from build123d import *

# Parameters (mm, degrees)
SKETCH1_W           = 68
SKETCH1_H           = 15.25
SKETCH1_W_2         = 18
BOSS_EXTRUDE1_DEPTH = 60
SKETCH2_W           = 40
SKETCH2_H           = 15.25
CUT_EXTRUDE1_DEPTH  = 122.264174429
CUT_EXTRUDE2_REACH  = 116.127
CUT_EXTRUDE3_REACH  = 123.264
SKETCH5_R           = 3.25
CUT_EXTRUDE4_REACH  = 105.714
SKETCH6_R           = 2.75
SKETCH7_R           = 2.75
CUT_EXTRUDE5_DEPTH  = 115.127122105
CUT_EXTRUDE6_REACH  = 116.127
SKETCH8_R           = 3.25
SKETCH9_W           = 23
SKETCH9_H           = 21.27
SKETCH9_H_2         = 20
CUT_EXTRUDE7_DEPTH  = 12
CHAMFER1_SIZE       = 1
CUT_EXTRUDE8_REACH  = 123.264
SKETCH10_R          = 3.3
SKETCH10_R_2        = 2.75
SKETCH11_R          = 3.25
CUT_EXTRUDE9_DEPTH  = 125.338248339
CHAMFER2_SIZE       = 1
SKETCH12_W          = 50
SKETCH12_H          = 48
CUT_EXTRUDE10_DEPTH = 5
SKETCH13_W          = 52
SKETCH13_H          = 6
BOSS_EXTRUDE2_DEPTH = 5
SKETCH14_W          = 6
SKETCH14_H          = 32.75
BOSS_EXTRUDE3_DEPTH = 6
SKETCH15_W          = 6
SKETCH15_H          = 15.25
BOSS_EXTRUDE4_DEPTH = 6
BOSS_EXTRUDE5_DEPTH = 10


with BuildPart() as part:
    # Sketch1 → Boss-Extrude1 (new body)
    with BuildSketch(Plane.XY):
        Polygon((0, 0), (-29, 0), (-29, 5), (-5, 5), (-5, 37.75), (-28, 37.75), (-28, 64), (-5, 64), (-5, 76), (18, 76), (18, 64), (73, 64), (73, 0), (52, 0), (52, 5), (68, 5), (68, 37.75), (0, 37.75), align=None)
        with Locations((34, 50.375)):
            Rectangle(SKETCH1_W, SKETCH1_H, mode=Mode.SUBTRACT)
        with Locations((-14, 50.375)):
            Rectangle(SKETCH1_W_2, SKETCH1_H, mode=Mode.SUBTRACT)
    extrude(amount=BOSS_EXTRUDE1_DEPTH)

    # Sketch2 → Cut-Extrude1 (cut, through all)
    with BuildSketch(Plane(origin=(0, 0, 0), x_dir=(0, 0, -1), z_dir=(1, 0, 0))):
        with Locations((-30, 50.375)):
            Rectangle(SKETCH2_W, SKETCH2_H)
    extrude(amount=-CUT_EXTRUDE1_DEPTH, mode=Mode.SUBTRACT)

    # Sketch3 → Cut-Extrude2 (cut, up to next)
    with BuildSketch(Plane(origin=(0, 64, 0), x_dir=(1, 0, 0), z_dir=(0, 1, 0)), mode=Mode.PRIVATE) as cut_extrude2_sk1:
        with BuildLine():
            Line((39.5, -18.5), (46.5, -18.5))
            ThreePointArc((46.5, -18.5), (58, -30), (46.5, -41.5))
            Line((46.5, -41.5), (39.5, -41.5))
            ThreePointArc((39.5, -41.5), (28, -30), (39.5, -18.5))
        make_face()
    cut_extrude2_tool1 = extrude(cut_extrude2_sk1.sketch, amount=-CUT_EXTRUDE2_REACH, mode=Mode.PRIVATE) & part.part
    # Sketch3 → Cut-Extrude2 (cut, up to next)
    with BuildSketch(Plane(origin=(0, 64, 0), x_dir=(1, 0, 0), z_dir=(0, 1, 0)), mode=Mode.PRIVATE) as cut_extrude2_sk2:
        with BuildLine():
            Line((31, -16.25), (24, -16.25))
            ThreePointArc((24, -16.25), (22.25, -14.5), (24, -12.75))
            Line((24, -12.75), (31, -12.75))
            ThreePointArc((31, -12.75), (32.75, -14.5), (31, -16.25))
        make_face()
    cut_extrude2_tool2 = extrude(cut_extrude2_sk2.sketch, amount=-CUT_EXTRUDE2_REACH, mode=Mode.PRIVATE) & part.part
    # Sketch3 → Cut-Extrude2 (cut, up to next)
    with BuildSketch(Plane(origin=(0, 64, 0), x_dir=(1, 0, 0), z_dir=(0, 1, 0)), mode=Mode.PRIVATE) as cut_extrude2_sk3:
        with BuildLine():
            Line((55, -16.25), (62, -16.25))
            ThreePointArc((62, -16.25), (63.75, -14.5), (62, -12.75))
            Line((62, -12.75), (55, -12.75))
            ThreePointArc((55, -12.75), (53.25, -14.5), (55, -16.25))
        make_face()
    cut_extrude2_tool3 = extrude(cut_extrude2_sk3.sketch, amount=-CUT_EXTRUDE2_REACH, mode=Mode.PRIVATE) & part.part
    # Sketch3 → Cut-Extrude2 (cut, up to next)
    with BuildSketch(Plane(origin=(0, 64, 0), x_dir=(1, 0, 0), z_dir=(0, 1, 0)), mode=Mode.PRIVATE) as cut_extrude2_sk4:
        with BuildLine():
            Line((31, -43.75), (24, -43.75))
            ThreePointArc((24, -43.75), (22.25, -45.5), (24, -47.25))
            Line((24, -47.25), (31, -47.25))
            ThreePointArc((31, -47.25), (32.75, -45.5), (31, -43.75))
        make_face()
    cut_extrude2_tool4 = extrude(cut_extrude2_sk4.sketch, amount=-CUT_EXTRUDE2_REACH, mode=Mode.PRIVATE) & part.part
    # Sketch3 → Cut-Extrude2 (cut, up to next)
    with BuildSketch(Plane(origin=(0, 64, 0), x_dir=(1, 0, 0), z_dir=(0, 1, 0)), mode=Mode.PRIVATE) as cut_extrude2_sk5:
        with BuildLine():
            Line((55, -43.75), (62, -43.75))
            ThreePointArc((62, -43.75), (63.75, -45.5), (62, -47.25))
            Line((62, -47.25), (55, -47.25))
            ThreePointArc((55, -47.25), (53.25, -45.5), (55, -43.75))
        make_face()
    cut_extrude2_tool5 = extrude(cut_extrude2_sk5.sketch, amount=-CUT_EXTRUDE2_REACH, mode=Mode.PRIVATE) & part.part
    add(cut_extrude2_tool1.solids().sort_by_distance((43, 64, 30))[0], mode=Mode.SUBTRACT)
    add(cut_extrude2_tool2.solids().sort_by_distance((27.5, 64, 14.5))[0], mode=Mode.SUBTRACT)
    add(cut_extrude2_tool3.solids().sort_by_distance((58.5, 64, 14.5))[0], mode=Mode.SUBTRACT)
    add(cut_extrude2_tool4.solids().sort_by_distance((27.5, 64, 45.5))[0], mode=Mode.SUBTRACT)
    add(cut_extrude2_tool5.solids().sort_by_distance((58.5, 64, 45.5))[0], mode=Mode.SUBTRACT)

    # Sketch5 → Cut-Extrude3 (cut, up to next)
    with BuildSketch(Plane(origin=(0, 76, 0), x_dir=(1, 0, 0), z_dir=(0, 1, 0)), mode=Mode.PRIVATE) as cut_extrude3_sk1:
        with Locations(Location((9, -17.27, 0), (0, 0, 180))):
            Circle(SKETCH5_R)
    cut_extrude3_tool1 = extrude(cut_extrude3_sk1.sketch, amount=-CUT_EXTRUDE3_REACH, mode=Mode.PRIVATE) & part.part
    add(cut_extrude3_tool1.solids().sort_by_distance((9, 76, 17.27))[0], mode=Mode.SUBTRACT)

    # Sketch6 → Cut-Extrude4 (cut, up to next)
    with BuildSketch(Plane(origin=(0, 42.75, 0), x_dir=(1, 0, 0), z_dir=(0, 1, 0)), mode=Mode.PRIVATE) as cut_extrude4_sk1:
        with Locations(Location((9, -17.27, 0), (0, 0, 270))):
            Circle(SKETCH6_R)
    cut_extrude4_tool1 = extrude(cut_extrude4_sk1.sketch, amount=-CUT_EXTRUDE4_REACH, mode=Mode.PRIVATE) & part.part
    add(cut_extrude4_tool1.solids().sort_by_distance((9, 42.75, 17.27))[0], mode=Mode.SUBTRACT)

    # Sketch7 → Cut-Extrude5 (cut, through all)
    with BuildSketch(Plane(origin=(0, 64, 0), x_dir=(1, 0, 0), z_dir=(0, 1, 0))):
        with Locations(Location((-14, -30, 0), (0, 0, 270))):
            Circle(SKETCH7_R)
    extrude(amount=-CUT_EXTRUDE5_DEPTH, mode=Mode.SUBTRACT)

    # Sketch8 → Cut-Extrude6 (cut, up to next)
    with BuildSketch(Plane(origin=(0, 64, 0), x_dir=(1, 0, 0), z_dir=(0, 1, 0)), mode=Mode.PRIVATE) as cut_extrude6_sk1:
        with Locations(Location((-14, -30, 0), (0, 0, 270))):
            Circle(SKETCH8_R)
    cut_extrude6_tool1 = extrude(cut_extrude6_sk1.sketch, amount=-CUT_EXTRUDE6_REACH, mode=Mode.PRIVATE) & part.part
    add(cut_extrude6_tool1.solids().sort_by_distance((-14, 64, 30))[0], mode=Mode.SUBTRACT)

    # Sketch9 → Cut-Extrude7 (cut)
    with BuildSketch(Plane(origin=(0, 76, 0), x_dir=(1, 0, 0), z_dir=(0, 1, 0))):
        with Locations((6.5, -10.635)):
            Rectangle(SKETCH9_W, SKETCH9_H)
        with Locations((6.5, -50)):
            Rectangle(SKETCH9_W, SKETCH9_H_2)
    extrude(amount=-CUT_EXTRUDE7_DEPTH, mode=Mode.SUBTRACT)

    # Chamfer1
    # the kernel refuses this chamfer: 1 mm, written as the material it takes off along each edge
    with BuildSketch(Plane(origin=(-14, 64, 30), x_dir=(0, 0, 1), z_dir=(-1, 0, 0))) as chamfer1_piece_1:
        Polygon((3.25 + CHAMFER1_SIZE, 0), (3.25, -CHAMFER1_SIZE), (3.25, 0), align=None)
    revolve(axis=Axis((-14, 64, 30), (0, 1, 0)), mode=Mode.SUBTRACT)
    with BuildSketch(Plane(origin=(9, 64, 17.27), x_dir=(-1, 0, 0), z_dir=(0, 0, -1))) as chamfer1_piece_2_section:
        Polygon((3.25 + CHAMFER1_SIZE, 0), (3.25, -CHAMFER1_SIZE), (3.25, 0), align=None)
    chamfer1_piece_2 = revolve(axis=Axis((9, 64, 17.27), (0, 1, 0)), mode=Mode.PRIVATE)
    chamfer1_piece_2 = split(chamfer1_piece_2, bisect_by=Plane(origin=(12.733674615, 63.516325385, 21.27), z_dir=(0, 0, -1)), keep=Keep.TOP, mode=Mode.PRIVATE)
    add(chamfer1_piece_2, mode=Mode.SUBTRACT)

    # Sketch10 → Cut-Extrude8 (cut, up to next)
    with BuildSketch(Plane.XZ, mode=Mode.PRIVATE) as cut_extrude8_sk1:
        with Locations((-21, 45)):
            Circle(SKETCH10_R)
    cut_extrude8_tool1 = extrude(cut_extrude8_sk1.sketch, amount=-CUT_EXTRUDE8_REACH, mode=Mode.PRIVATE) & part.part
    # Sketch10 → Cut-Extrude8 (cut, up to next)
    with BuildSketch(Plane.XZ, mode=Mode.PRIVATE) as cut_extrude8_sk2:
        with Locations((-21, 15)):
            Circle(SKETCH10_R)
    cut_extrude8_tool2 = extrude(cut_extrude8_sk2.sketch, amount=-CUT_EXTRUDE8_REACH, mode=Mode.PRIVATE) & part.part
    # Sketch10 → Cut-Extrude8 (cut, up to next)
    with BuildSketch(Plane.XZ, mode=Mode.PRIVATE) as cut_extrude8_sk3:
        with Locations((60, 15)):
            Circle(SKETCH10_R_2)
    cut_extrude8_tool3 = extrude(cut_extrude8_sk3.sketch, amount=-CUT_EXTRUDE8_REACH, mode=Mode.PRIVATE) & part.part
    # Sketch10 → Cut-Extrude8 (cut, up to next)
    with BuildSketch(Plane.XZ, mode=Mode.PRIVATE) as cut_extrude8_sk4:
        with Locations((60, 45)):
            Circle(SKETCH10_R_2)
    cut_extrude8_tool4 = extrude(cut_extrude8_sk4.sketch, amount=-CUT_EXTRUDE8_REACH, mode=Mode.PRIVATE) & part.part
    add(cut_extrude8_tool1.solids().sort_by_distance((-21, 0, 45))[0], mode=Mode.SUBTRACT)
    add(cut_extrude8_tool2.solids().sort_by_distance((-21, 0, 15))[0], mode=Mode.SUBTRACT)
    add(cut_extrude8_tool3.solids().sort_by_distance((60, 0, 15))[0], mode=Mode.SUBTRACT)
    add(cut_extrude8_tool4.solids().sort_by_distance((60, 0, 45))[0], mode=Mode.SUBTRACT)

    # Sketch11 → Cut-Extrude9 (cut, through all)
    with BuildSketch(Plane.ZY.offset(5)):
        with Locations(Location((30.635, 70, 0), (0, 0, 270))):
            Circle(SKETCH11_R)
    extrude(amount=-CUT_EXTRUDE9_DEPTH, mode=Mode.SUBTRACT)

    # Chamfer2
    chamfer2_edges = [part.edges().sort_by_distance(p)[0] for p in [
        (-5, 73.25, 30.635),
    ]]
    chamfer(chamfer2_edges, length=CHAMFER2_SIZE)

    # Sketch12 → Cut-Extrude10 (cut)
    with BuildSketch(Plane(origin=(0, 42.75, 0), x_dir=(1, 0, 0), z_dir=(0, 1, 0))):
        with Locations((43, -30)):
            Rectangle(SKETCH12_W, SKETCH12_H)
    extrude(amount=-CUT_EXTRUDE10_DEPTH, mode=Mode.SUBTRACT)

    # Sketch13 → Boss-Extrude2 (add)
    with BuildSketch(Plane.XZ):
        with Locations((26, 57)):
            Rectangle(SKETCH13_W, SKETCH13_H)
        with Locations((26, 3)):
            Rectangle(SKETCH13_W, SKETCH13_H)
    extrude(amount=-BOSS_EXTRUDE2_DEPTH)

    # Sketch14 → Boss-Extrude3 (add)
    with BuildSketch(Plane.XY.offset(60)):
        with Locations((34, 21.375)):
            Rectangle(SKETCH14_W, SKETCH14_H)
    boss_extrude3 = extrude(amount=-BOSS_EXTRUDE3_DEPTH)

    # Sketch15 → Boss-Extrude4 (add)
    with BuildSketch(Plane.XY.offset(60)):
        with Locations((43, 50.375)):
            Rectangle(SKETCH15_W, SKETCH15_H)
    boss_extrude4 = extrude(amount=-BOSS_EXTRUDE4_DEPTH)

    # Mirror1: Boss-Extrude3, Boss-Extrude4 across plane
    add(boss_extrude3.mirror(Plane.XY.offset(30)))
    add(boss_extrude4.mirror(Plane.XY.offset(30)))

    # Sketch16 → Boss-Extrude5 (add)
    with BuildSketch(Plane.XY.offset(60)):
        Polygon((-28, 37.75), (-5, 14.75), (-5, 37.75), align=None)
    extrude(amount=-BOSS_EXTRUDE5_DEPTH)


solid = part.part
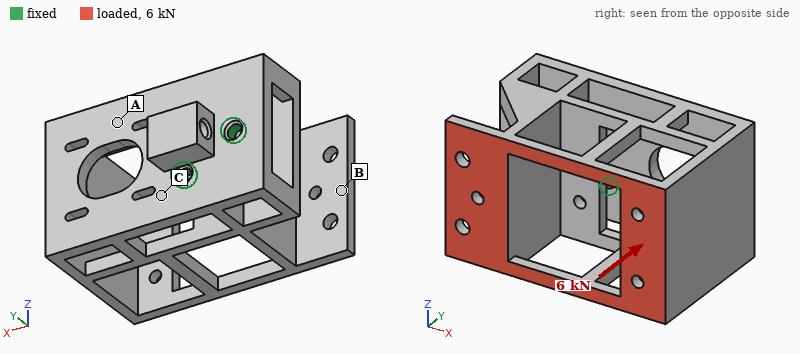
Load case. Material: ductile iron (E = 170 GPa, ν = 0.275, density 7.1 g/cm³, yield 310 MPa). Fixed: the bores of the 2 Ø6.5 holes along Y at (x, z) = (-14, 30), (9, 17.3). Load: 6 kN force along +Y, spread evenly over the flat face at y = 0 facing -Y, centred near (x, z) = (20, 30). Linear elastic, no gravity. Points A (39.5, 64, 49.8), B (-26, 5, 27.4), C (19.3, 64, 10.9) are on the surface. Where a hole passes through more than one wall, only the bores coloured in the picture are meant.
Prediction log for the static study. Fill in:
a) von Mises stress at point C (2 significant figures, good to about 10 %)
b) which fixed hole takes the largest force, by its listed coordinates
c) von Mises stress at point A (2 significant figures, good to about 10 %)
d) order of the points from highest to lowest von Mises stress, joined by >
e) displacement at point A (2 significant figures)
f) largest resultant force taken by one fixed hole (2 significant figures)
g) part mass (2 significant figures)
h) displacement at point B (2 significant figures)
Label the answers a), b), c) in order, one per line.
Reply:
a) 130 MPa
b) (9, 17.3)
c) 53 MPa
d) C > A > B
e) 0.24 mm
f) 5.8 kN
g) 740 g
h) 0.23 mm
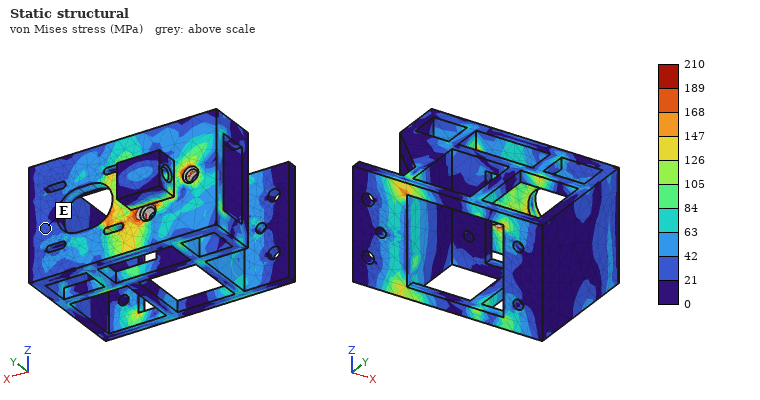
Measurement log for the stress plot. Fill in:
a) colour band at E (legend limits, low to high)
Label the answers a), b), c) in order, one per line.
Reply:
a) 21 to 42 MPa
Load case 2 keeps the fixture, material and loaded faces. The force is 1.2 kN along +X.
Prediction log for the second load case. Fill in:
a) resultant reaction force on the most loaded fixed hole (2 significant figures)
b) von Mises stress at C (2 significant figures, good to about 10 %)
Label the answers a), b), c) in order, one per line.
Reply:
a) 1.9 kN
b) 44 MPa
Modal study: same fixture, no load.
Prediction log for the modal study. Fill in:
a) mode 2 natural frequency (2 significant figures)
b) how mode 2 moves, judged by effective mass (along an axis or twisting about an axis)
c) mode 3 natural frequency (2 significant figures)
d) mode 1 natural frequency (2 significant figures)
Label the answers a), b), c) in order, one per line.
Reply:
a) 880 Hz
b) along Z
c) 1600 Hz
d) 610 Hz
